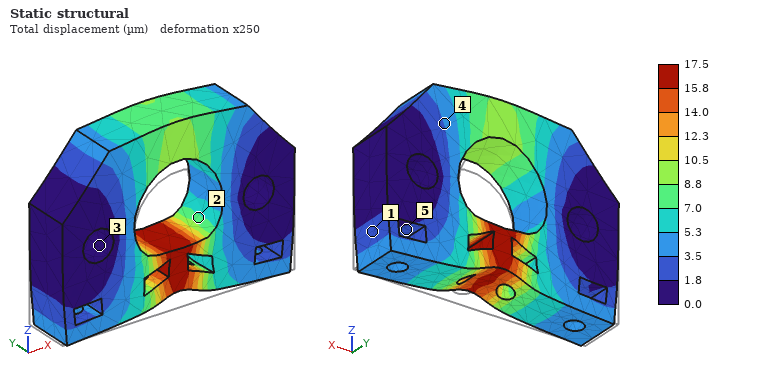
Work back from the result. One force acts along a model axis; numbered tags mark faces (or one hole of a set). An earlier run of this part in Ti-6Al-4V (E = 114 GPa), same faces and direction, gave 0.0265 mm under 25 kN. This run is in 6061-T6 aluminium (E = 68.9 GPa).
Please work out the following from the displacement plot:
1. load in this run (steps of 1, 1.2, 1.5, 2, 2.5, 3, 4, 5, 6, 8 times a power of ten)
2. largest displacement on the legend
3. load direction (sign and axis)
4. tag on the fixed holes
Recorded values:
10 kN
17.5 µm
+Z
3
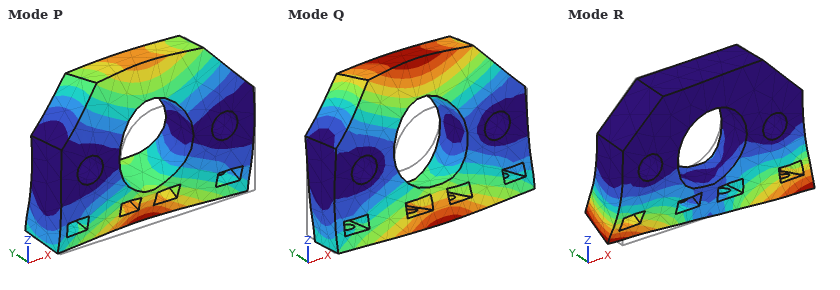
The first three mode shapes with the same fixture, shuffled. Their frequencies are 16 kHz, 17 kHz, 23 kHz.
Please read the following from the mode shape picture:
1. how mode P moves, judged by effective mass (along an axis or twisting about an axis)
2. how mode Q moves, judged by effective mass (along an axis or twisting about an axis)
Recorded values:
along Y
twisting about X
